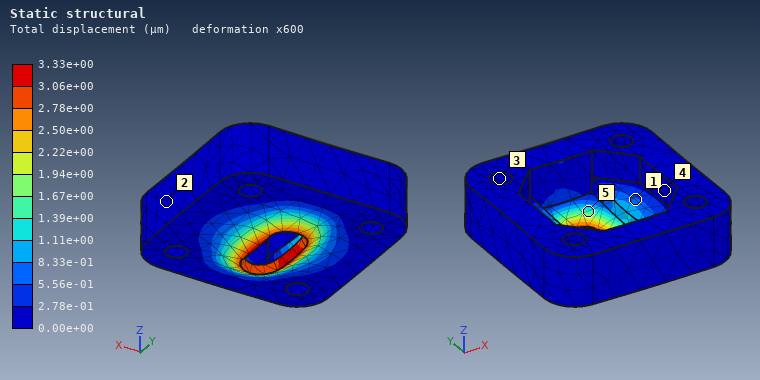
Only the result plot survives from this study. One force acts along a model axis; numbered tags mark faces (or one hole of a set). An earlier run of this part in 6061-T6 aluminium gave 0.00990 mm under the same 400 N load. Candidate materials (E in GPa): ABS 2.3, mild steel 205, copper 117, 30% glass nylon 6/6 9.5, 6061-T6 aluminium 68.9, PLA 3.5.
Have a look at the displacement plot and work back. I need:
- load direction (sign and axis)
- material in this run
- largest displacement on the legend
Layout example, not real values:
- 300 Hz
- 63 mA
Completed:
- -Z
- mild steel
- 3.33e+00 µm
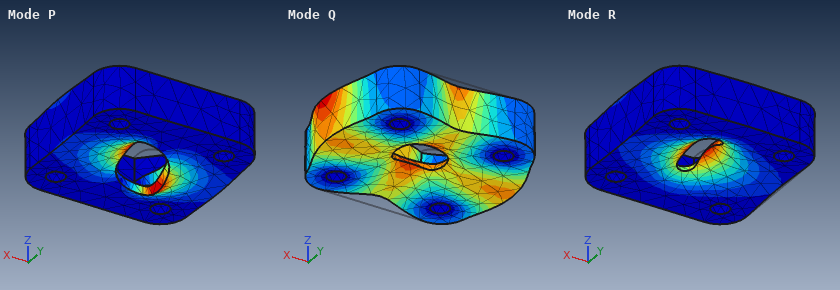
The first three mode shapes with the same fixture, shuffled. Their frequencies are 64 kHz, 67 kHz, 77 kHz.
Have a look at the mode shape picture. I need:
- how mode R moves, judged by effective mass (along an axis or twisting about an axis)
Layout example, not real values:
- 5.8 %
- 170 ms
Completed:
- along Z
